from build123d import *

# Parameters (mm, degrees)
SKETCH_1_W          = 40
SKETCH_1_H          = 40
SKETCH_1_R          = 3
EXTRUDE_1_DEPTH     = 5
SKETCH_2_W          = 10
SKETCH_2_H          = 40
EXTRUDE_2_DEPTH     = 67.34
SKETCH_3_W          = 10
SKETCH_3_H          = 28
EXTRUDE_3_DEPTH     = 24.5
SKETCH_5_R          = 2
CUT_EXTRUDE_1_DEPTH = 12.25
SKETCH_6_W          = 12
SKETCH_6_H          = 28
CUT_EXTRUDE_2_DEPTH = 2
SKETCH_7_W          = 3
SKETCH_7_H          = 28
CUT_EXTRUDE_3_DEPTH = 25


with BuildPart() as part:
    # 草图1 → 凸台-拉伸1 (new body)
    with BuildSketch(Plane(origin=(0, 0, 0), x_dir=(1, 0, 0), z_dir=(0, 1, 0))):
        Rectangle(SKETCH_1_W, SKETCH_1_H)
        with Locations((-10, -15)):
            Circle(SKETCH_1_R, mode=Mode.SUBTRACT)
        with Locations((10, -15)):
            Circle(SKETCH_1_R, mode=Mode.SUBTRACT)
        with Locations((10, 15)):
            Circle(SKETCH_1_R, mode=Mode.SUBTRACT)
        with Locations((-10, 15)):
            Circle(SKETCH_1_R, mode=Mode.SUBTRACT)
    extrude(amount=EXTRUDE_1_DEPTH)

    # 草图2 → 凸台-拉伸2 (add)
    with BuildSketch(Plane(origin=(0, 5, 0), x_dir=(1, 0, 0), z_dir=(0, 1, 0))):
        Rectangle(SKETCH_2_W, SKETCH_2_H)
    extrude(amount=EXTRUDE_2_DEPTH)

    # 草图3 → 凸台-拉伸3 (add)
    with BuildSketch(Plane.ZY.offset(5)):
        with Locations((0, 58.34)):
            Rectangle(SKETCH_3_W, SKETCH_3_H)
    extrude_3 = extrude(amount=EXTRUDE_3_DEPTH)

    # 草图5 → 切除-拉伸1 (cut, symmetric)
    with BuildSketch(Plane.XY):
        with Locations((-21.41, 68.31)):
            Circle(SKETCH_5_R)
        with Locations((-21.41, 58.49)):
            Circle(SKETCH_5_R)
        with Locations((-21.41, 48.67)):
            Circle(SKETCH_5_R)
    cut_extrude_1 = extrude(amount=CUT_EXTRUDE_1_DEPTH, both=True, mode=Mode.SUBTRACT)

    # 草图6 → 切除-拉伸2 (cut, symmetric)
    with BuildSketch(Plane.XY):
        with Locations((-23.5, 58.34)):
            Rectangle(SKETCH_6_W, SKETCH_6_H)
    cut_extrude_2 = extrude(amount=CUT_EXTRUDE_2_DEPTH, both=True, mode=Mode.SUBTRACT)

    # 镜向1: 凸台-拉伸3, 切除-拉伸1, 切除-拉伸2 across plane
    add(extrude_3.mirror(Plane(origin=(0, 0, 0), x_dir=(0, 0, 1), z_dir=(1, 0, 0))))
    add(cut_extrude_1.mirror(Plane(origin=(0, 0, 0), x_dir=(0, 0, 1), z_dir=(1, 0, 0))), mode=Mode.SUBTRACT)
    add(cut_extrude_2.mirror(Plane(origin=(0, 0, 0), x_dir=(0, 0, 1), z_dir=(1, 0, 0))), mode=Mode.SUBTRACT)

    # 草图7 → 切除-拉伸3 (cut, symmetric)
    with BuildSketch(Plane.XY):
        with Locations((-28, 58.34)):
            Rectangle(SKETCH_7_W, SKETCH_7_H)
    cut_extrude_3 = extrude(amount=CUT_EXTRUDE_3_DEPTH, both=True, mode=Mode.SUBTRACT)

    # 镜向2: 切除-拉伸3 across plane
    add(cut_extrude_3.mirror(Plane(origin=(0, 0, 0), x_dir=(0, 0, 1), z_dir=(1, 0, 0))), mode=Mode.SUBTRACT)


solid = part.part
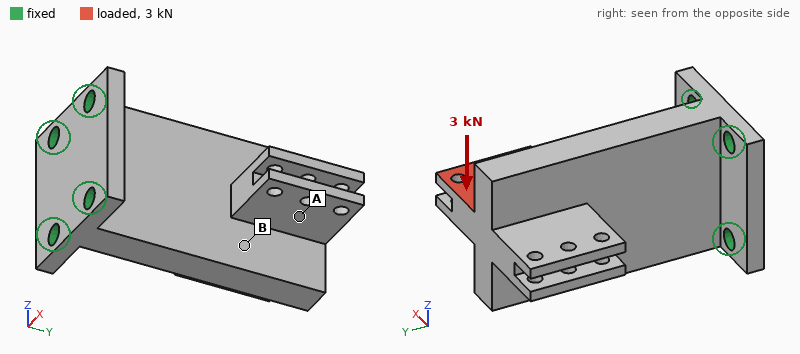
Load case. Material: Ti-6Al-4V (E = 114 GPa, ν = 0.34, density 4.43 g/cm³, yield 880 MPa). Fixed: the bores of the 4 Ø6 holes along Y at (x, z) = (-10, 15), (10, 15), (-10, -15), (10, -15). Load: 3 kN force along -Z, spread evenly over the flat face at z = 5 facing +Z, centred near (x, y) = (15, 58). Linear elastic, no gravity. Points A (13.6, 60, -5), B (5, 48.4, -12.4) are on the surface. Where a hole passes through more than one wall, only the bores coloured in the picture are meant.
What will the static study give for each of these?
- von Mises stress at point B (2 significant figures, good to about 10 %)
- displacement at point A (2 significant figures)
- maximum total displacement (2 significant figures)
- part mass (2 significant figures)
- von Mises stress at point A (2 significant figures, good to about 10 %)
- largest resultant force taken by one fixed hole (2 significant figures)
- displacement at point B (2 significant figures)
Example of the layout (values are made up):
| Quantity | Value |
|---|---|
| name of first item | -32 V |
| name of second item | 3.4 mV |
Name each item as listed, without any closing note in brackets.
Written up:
| Quantity | Value |
|---|---|
| von Mises stress at point B | 53 MPa |
| displacement at point A | 0.13 mm |
| maximum total displacement | 0.24 mm |
| part mass | 190 g |
| von Mises stress at point A | 17 MPa |
| largest resultant force taken by one fixed hole | 4.0 kN |
| displacement at point B | 0.078 mm |
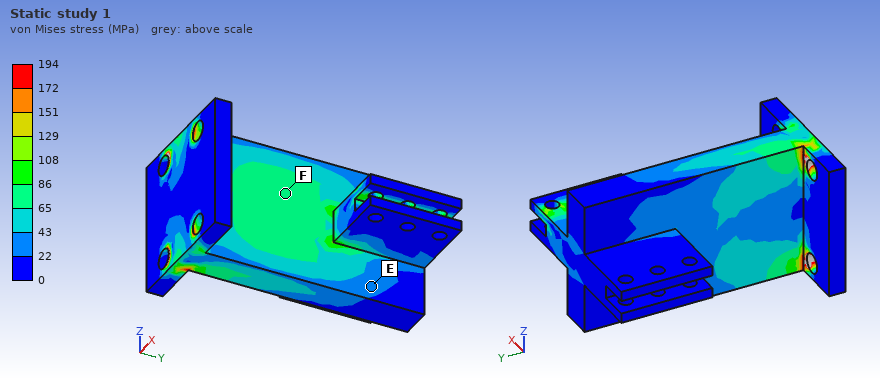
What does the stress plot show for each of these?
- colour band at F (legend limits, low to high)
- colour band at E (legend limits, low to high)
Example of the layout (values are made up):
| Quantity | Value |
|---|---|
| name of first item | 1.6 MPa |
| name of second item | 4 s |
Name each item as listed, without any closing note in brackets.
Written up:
| Quantity | Value |
|---|---|
| colour band at F | 65 to 86 MPa |
| colour band at E | 22 to 43 MPa |
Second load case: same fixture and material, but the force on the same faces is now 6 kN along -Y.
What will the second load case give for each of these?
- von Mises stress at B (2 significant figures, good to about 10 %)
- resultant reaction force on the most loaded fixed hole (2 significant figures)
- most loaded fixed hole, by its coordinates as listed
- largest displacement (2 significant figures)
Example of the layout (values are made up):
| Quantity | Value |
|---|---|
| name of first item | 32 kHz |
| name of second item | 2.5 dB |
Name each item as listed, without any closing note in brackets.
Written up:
| Quantity | Value |
|---|---|
| von Mises stress at B | 88 MPa |
| resultant reaction force on the most loaded fixed hole | 5.1 kN |
| most loaded fixed hole, by its coordinates as listed | (10, 15) |
| largest displacement | 0.68 mm |
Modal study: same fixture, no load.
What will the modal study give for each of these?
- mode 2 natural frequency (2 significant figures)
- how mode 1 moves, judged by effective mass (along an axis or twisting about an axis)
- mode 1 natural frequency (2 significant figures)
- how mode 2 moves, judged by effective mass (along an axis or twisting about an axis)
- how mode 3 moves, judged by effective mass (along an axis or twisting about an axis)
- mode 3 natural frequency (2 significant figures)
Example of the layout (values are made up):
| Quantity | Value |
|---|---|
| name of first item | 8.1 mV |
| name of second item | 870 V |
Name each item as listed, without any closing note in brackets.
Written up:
| Quantity | Value |
|---|---|
| mode 2 natural frequency | 3300 Hz |
| how mode 1 moves, judged by effective mass | along X |
| mode 1 natural frequency | 1100 Hz |
| how mode 2 moves, judged by effective mass | along Z |
| how mode 3 moves, judged by effective mass | twisting about Y |
| mode 3 natural frequency | 3900 Hz |
